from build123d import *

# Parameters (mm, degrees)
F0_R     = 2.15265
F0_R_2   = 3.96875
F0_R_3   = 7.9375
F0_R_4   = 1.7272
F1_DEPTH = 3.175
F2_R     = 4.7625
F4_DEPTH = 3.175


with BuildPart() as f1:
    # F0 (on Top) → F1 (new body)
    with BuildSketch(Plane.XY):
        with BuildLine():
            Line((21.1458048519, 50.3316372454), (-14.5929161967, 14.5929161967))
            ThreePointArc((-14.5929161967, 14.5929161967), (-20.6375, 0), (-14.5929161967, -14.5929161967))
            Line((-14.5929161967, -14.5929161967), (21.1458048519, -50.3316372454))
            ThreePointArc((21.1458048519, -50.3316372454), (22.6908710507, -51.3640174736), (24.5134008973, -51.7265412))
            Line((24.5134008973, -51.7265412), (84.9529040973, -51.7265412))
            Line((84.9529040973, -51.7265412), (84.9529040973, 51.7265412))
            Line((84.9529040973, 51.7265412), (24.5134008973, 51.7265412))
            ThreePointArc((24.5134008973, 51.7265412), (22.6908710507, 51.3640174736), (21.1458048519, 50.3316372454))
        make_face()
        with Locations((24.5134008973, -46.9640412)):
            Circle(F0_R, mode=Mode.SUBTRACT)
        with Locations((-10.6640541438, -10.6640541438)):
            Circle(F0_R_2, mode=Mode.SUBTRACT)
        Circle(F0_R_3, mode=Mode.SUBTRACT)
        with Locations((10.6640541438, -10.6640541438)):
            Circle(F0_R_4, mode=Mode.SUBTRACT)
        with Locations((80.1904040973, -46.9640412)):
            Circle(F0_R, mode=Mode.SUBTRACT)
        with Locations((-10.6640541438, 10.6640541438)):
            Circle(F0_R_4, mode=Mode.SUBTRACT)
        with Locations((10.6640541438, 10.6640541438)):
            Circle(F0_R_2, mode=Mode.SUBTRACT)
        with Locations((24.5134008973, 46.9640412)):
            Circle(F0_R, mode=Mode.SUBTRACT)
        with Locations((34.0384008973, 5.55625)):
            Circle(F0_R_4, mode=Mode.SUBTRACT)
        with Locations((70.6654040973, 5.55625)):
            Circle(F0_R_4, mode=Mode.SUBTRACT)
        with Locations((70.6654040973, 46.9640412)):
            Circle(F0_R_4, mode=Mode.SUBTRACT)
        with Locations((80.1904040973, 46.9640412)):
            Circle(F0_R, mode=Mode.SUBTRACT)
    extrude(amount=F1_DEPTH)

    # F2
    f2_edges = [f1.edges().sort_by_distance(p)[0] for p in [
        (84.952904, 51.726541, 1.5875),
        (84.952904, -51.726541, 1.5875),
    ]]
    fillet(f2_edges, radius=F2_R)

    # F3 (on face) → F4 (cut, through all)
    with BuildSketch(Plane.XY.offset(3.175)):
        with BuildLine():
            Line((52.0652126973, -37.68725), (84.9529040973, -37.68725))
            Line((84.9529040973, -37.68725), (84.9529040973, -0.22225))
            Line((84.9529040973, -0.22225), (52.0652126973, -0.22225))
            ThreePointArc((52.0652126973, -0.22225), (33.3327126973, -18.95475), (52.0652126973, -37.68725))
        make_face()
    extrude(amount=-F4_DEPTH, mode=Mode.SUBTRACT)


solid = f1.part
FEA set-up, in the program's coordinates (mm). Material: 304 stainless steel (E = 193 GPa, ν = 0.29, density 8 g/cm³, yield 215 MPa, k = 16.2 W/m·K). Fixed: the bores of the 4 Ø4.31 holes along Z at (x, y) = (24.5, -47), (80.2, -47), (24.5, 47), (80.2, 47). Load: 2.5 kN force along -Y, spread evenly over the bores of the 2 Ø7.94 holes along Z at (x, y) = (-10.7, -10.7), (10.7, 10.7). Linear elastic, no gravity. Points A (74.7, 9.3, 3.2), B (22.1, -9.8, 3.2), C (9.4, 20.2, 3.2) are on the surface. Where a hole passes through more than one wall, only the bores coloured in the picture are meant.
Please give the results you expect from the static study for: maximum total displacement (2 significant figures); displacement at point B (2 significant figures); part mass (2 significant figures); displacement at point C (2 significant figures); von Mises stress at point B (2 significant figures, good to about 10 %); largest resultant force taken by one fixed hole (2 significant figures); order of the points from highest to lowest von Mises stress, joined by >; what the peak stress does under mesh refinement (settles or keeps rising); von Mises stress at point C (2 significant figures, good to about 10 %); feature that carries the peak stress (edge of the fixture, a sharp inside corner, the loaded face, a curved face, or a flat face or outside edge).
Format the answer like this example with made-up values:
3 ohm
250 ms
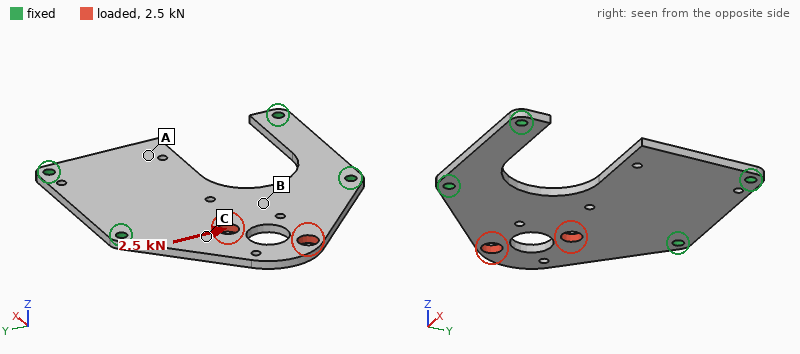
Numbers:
11 µm
2.6 µm
170 g
4.2 µm
10 MPa
1.3 kN
C > B > A
keeps rising
19 MPa
edge of the fixture
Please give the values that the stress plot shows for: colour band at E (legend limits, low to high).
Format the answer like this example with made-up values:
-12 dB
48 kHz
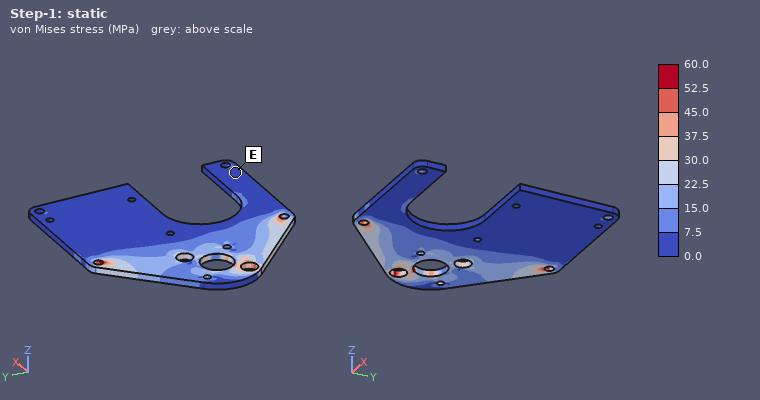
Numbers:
0.0 to 7.5 MPa
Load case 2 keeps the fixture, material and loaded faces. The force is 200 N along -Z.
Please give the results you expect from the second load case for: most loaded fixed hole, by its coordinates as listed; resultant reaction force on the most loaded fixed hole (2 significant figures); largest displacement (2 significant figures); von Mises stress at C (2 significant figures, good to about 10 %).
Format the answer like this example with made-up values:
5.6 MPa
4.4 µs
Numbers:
(24.5, 47)
130 N
0.21 mm
21 MPa
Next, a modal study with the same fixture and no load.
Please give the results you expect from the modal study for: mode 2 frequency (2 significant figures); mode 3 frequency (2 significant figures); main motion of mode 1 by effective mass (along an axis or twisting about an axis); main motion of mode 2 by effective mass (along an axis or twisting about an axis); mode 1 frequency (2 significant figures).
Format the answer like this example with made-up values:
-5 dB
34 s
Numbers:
1400 Hz
2700 Hz
along Z
along Z
1100 Hz
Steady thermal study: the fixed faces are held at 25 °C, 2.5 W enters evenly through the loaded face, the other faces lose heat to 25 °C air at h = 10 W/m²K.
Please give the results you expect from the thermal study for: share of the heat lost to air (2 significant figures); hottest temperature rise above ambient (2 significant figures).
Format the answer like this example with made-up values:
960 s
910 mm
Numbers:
51 %
36 K
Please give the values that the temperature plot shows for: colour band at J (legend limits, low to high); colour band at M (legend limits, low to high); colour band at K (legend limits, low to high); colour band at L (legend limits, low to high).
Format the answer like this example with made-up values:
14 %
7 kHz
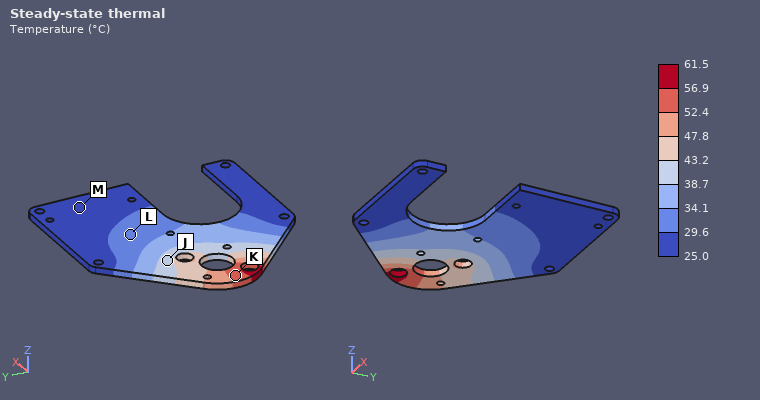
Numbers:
38.7 to 43.2 °C
25.0 to 29.6 °C
52.4 to 56.9 °C
29.6 to 34.1 °C
